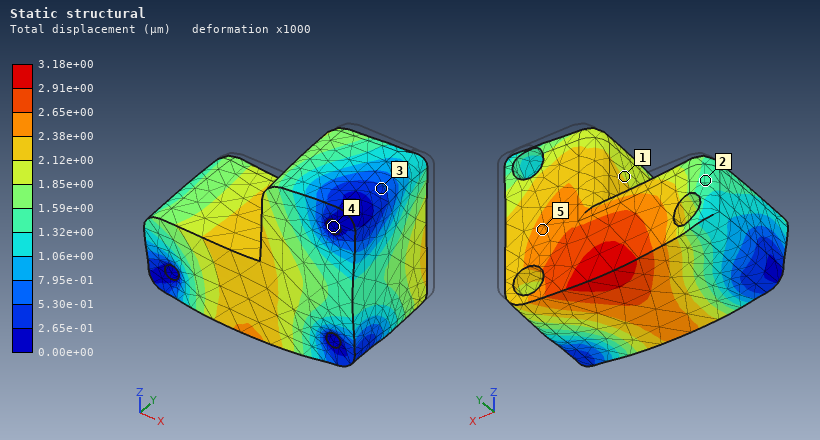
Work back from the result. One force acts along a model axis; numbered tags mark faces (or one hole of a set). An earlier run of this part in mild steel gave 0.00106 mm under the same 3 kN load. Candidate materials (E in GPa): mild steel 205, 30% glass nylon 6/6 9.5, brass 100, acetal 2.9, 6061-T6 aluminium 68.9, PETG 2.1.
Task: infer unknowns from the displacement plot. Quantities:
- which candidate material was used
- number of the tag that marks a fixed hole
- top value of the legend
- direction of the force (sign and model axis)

6061-T6 aluminium
4
3.18e+00 µm
-Y
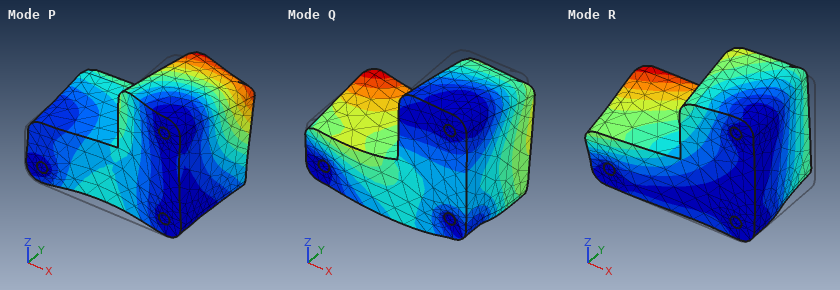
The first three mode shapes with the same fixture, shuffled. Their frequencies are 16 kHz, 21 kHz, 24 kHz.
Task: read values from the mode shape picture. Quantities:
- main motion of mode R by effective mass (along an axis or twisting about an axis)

along Z
